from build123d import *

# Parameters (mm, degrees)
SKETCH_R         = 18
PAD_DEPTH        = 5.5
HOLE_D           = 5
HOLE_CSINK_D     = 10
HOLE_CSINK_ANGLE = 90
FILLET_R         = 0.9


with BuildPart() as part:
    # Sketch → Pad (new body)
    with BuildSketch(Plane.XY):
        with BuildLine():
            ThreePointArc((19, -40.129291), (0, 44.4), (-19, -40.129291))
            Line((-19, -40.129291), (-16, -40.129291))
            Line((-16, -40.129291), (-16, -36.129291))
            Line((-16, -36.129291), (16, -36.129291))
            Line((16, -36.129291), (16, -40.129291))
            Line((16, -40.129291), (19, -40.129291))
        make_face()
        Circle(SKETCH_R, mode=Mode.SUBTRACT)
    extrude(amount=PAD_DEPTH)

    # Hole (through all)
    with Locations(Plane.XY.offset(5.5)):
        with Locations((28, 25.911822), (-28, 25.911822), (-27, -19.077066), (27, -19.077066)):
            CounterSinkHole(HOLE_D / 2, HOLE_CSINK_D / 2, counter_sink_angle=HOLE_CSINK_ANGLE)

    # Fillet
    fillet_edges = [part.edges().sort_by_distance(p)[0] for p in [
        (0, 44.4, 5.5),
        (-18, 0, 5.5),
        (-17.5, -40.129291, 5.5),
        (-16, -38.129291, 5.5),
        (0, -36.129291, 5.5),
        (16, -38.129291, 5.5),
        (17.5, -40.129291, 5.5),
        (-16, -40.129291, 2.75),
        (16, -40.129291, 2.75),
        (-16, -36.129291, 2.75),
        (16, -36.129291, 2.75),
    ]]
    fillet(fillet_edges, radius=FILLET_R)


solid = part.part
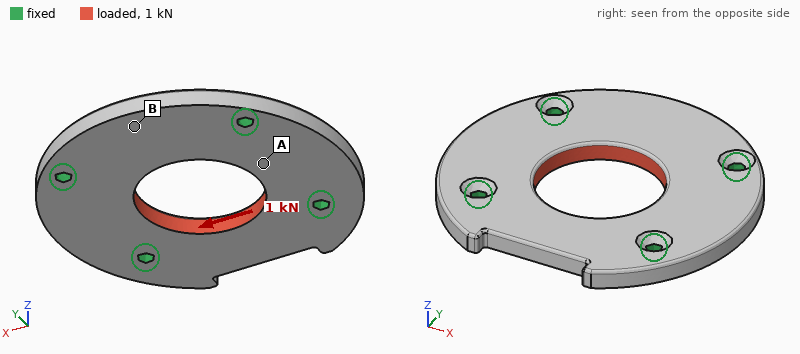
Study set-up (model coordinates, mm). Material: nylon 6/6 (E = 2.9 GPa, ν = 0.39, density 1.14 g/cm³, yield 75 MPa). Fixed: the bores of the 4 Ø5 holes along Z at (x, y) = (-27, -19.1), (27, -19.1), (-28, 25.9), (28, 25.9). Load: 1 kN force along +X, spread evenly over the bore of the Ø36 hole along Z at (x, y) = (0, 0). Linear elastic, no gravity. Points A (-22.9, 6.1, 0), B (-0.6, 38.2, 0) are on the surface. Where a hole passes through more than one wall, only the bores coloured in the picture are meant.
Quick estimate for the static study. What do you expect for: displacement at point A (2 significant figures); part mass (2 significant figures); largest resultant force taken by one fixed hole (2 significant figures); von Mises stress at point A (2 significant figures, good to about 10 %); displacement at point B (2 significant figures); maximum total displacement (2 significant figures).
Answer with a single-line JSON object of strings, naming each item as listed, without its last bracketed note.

{"displacement at point A": "24 µm", "part mass": "30 g", "largest resultant force taken by one fixed hole": "270 N", "von Mises stress at point A": "1.7 MPa", "displacement at point B": "9.2 µm", "maximum total displacement": "28 µm"}
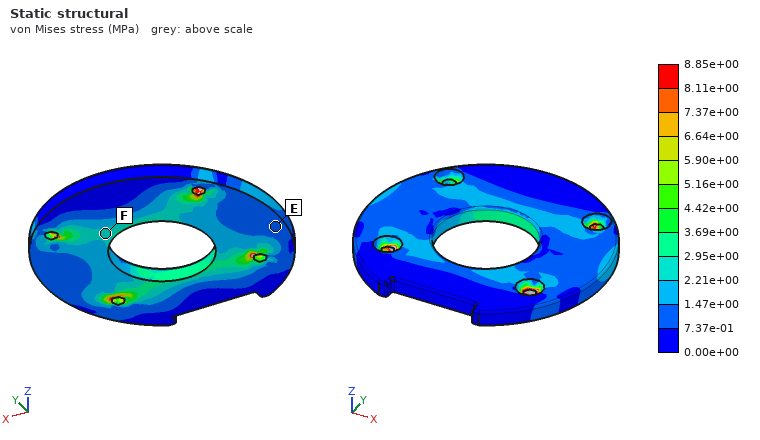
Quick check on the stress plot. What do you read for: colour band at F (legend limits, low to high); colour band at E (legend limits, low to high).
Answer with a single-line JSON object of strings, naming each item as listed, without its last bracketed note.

{"colour band at F": "2.21e+00 to 2.95e+00 MPa", "colour band at E": "7.37e-01 to 1.47e+00 MPa"}
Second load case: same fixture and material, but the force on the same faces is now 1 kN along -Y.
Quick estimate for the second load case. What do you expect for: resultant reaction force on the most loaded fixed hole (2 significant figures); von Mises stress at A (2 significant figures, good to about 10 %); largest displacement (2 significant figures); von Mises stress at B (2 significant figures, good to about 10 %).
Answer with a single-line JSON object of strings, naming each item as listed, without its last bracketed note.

{"resultant reaction force on the most loaded fixed hole": "270 N", "von Mises stress at A": "2.4 MPa", "largest displacement": "46 µm", "von Mises stress at B": "1.3 MPa"}
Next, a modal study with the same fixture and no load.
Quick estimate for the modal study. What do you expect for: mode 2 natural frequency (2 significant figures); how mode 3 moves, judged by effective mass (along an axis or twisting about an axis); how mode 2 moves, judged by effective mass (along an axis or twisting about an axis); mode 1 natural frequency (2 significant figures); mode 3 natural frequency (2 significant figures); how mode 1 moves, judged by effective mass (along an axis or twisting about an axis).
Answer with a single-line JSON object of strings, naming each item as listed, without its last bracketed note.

{"mode 2 natural frequency": "2100 Hz", "how mode 3 moves, judged by effective mass": "twisting about Y", "how mode 2 moves, judged by effective mass": "twisting about X", "mode 1 natural frequency": "1900 Hz", "mode 3 natural frequency": "2800 Hz", "how mode 1 moves, judged by effective mass": "along Z"}
